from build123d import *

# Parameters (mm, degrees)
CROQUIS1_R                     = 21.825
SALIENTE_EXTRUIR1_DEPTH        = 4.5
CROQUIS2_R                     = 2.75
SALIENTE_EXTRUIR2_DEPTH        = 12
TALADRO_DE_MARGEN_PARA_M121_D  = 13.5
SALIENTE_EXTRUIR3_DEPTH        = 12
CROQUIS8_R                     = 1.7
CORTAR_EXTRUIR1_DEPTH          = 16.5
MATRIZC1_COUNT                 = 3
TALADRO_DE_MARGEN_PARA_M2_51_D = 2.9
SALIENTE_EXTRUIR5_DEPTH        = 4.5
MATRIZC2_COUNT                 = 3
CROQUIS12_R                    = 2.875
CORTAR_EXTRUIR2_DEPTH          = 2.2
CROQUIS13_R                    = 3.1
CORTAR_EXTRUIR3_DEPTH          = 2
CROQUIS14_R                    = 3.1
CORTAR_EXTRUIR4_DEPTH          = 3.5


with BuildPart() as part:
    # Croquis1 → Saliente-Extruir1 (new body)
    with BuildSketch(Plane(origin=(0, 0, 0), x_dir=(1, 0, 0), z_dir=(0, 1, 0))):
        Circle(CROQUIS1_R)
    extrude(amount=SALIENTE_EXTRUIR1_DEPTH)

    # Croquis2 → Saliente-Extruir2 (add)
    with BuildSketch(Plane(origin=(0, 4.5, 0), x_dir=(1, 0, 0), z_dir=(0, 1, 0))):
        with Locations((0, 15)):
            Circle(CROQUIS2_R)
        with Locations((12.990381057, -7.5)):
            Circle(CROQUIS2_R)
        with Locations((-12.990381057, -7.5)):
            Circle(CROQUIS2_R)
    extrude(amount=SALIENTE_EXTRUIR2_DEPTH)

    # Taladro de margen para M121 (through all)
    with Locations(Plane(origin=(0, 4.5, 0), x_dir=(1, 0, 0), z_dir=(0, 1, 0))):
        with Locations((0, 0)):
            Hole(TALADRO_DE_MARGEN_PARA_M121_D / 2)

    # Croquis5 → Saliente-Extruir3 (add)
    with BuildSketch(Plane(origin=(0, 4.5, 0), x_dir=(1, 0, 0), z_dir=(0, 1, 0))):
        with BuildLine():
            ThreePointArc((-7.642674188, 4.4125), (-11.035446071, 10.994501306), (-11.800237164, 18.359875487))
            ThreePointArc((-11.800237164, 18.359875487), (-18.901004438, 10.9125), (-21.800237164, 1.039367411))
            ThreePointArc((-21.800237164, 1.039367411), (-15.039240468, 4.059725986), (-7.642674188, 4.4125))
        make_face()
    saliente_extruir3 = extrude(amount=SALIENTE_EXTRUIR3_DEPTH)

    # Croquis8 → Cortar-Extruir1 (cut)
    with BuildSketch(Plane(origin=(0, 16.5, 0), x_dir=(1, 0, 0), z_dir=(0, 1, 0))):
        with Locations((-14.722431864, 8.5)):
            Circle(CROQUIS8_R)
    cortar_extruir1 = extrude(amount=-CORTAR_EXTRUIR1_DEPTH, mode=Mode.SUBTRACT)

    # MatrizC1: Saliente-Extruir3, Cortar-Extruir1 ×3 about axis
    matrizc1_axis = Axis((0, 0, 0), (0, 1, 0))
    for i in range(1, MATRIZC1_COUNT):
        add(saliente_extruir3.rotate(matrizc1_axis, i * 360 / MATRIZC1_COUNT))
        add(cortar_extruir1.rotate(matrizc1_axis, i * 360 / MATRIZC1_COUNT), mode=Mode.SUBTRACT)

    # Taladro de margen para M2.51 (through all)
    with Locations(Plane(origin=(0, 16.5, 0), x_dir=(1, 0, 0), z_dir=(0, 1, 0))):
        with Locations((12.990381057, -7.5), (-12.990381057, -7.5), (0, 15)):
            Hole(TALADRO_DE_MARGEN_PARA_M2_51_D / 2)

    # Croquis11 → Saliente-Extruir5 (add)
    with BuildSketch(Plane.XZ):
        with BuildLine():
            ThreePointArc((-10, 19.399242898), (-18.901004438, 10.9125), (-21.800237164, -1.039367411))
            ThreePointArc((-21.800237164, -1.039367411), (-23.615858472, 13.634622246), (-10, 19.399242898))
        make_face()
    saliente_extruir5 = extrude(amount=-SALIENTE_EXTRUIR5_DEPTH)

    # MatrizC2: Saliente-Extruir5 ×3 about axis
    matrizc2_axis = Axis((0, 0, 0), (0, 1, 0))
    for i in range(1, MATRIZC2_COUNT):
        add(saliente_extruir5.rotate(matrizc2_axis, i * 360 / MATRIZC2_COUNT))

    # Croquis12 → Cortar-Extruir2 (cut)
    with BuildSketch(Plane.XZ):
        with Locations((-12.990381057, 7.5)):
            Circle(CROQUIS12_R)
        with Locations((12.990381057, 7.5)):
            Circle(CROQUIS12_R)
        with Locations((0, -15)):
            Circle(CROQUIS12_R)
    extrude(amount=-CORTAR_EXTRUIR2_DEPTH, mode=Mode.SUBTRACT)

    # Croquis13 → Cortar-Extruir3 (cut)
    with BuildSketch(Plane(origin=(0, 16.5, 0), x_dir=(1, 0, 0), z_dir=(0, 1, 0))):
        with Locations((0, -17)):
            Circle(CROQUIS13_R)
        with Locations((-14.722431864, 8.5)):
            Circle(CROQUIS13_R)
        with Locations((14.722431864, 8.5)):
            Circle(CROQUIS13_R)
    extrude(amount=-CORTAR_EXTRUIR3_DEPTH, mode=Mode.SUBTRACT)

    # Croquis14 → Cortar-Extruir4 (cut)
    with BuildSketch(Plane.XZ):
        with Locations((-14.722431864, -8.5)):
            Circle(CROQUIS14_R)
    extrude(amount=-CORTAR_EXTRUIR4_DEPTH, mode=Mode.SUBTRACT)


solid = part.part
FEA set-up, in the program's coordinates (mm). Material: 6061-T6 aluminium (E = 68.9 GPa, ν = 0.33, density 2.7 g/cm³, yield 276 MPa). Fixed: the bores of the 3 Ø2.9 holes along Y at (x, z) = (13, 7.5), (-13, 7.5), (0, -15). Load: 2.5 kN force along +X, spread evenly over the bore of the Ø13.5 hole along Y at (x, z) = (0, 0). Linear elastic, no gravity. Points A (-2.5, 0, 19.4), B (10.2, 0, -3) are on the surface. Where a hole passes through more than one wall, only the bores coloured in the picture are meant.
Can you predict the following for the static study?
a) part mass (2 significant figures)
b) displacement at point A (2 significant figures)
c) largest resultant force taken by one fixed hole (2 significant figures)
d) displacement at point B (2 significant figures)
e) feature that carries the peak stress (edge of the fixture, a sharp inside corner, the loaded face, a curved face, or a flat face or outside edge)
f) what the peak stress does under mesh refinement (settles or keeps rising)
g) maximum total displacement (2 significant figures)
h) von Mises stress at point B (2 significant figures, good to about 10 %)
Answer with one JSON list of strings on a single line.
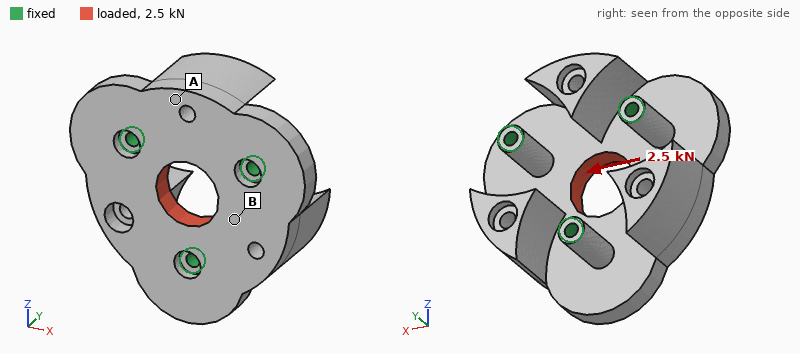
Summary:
["30 g", "1.3 µm", "840 N", "5.1 µm", "edge of the fixture", "keeps rising", "6.4 µm", "11 MPa"]
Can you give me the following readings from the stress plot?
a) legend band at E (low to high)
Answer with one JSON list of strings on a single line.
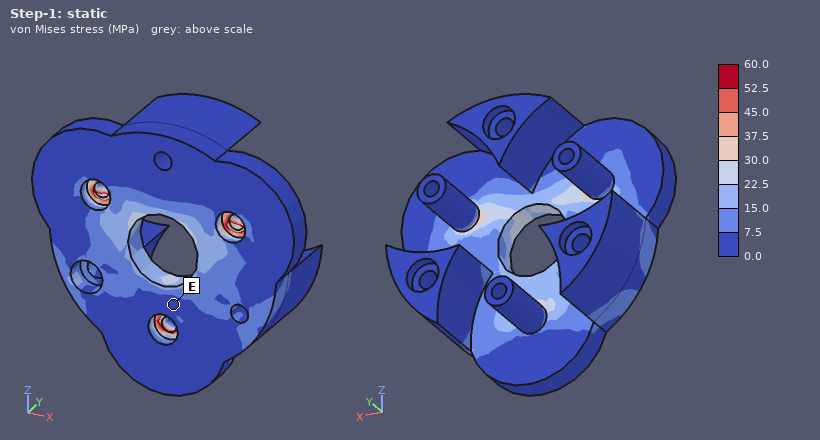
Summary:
["0.0 to 7.5 MPa"]
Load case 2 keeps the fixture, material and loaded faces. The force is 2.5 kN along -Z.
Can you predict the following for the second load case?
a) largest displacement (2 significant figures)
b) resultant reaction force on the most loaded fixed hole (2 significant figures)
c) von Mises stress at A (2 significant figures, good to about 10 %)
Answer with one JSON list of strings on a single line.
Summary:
["7.3 µm", "840 N", "12 MPa"]
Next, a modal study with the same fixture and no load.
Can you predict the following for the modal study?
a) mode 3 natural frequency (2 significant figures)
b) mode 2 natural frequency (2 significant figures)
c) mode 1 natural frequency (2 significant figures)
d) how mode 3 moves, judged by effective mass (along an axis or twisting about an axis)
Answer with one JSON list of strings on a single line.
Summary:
["8900 Hz", "7300 Hz", "7300 Hz", "along Y"]
